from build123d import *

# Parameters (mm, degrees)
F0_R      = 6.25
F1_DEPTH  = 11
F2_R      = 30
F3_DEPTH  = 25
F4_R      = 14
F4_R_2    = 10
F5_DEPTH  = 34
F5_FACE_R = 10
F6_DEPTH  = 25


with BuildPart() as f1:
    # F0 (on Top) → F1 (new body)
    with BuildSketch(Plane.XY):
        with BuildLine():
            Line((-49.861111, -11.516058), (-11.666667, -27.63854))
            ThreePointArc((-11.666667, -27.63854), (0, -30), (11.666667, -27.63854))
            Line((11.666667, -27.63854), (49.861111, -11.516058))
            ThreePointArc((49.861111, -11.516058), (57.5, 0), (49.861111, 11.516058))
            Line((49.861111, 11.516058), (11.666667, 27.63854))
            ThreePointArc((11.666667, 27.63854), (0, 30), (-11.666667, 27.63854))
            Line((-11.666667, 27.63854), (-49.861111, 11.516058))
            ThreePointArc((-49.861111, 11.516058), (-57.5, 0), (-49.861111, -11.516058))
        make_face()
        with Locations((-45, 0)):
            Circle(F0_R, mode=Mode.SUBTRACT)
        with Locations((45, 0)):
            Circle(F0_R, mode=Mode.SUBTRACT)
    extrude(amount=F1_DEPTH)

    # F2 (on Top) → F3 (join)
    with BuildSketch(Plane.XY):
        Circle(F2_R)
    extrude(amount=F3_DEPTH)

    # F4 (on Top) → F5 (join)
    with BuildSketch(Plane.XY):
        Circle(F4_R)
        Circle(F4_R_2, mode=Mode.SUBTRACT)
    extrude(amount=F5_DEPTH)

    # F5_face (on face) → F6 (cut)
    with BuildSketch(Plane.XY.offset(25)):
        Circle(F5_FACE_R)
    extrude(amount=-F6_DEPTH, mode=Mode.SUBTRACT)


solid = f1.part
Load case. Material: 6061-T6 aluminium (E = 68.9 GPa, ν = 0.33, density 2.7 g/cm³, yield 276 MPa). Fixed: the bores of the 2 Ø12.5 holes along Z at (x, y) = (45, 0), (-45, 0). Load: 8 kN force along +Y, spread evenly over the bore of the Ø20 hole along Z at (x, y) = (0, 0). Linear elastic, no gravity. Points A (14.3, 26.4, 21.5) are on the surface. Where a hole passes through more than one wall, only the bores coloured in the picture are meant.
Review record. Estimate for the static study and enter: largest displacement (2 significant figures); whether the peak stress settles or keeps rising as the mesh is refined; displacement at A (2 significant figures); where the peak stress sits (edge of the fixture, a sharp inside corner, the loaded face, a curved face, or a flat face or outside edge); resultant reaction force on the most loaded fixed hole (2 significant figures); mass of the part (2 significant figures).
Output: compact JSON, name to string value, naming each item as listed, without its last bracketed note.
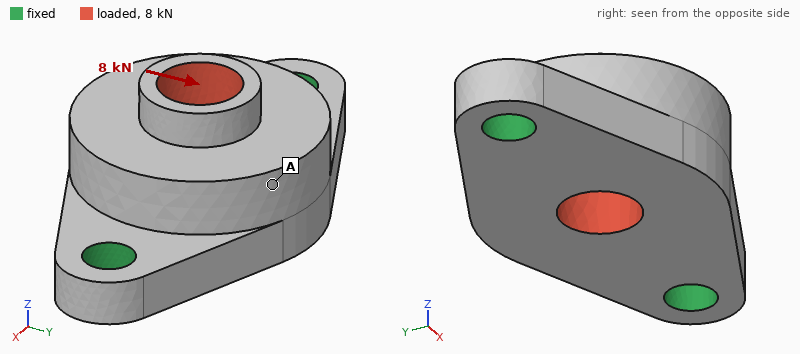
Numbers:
{"largest displacement": "77 µm", "whether the peak stress settles or keeps rising as the mesh is refined": "keeps rising", "displacement at A": "65 µm", "where the peak stress sits": "edge of the fixture", "resultant reaction force on the most loaded fixed hole": "4.0 kN", "mass of the part": "220 g"}
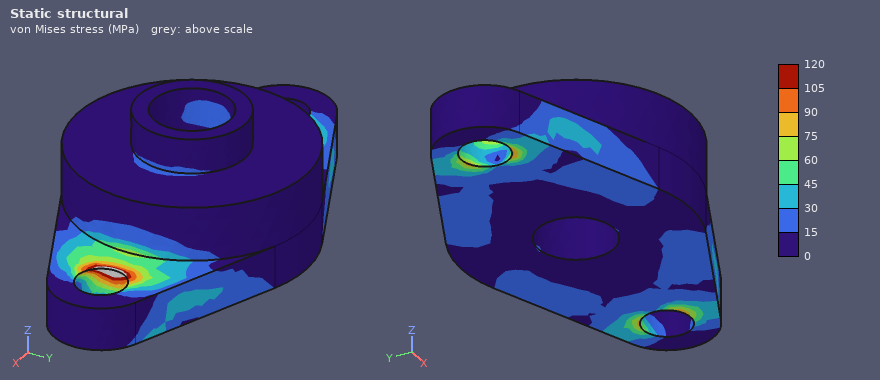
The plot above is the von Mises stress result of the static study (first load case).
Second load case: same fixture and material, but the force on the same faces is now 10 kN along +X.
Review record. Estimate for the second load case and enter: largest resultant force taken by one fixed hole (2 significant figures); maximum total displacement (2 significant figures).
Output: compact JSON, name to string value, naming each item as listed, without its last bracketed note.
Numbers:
{"largest resultant force taken by one fixed hole": "5.3 kN", "maximum total displacement": "17 µm"}
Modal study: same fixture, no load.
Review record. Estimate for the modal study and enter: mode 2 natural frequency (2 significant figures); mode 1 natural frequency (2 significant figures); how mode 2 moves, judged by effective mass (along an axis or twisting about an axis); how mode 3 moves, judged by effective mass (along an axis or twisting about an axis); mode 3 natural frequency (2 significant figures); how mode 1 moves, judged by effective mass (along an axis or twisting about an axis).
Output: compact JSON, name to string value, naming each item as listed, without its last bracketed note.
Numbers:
{"mode 2 natural frequency": "6800 Hz", "mode 1 natural frequency": "4200 Hz", "how mode 2 moves, judged by effective mass": "along Z", "how mode 3 moves, judged by effective mass": "along Y", "mode 3 natural frequency": "11 kHz", "how mode 1 moves, judged by effective mass": "along Y"}
